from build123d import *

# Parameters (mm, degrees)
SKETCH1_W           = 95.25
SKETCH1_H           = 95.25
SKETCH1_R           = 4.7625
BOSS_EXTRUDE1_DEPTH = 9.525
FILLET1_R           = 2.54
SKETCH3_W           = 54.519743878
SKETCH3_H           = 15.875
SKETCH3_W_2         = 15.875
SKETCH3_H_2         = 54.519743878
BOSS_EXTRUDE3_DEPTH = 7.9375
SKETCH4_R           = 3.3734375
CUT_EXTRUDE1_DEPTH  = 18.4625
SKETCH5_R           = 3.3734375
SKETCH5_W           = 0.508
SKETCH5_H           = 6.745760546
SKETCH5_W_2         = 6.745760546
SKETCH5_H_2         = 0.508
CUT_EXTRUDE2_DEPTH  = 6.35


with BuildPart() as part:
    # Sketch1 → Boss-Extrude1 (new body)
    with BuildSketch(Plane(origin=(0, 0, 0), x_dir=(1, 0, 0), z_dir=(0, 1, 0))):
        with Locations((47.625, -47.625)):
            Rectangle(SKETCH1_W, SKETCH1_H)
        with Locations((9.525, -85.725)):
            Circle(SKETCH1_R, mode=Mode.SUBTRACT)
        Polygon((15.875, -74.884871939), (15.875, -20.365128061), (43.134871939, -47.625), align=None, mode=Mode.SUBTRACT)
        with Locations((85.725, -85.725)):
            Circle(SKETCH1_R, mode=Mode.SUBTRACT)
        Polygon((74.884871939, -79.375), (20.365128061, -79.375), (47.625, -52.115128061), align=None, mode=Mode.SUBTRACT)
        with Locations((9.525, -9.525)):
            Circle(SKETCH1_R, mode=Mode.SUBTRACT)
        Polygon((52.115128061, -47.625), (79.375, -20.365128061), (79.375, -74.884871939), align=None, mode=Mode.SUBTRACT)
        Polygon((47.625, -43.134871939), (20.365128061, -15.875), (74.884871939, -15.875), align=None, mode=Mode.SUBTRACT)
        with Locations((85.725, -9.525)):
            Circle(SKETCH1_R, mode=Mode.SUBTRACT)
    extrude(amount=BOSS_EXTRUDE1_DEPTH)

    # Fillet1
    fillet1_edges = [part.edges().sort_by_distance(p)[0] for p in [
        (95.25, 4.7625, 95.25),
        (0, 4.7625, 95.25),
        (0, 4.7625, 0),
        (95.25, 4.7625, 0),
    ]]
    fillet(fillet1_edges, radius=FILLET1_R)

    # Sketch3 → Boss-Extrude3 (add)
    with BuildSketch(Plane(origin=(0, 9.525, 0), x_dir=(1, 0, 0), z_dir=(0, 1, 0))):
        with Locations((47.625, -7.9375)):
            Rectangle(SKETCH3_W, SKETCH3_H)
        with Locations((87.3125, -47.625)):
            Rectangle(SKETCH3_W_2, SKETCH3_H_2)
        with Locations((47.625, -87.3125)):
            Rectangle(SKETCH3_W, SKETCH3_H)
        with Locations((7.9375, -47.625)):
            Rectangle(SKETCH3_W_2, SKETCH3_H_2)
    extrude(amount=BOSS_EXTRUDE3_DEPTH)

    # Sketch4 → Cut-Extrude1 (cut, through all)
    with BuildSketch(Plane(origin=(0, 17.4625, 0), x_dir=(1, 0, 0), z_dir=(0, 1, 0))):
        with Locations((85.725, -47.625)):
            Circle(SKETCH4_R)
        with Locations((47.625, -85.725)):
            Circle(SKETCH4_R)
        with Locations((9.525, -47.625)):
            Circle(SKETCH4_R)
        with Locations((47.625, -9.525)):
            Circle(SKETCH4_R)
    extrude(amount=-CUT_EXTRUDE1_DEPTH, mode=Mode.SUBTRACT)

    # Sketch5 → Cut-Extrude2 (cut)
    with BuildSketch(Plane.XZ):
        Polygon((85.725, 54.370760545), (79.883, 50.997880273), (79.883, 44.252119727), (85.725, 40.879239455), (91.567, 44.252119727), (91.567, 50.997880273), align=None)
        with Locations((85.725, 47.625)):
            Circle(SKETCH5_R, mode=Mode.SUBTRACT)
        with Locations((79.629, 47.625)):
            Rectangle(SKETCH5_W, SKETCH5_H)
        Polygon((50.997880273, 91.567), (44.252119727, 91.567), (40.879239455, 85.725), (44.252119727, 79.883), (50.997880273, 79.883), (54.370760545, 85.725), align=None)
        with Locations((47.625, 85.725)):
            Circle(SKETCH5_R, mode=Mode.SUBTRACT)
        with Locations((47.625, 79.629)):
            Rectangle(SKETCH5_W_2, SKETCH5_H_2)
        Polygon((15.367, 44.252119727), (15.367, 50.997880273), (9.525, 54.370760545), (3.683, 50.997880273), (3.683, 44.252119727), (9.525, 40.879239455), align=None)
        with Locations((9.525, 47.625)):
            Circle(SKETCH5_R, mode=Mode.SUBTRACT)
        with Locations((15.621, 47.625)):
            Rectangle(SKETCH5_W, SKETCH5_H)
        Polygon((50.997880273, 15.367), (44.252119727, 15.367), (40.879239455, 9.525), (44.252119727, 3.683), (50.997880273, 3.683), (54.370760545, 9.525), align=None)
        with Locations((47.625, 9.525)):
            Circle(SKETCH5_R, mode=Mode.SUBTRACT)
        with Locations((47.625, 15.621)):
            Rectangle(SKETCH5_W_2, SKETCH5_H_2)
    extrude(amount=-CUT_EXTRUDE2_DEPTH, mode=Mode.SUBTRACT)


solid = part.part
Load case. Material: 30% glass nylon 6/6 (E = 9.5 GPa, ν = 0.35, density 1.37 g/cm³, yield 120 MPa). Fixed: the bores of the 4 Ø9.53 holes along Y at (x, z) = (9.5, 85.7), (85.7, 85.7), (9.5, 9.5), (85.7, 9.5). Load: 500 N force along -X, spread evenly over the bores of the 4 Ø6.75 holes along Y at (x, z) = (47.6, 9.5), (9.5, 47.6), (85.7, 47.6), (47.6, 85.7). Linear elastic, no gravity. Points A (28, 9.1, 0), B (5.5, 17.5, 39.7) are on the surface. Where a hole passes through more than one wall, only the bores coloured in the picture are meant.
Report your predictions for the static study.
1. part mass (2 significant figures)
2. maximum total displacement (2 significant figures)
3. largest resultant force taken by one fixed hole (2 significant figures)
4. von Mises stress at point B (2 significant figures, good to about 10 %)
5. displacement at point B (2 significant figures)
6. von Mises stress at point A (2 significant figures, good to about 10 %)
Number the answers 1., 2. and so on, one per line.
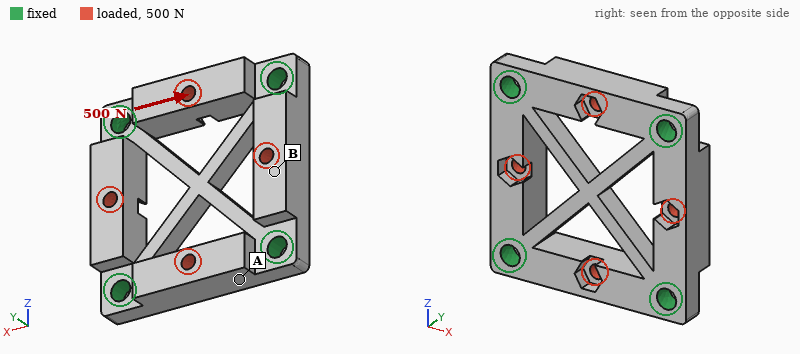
1. 110 g
2. 14 µm
3. 130 N
4. 1.0 MPa
5. 12 µm
6. 0.47 MPa
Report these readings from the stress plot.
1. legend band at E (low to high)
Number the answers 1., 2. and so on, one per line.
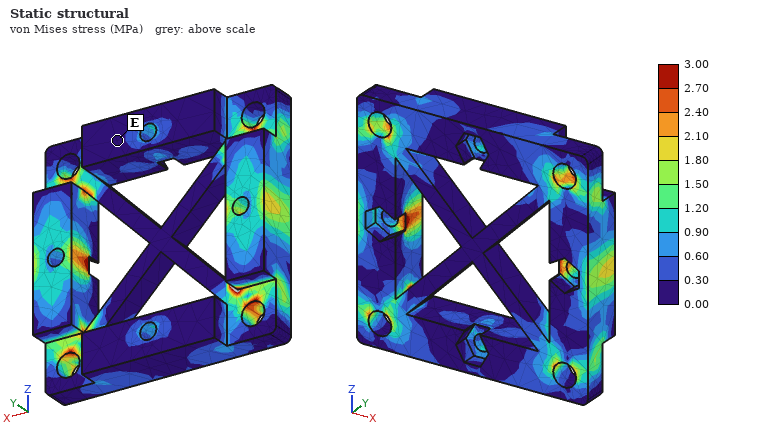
1. 0.00 to 0.30 MPa
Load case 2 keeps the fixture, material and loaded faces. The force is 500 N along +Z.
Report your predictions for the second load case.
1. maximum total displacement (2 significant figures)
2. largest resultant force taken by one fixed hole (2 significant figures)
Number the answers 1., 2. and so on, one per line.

1. 14 µm
2. 130 N
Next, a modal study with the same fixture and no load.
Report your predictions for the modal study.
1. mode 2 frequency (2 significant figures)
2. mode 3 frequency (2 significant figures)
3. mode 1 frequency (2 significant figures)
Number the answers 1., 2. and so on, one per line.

1. 4900 Hz
2. 5300 Hz
3. 3000 Hz
